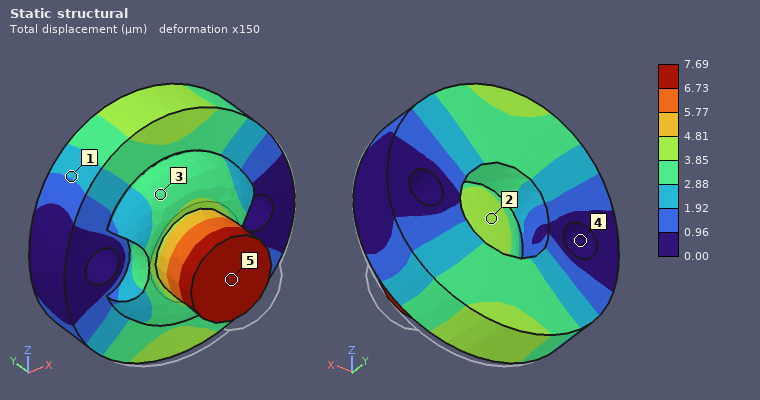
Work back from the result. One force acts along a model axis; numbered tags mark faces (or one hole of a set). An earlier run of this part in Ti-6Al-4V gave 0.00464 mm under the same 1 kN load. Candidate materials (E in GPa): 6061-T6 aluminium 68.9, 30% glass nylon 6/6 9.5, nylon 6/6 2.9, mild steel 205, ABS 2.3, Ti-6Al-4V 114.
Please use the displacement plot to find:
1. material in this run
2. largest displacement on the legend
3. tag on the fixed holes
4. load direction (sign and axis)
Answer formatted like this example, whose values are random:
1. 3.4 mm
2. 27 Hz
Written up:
1. 6061-T6 aluminium
2. 7.69 µm
3. 4
4. +Y
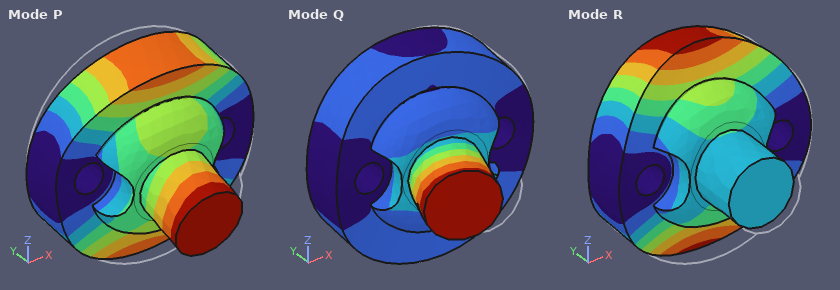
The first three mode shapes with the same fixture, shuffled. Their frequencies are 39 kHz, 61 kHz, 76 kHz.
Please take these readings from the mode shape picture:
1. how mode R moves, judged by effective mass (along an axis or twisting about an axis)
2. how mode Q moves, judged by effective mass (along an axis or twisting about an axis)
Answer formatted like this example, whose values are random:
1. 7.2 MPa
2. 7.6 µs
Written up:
1. along Y
2. along X
